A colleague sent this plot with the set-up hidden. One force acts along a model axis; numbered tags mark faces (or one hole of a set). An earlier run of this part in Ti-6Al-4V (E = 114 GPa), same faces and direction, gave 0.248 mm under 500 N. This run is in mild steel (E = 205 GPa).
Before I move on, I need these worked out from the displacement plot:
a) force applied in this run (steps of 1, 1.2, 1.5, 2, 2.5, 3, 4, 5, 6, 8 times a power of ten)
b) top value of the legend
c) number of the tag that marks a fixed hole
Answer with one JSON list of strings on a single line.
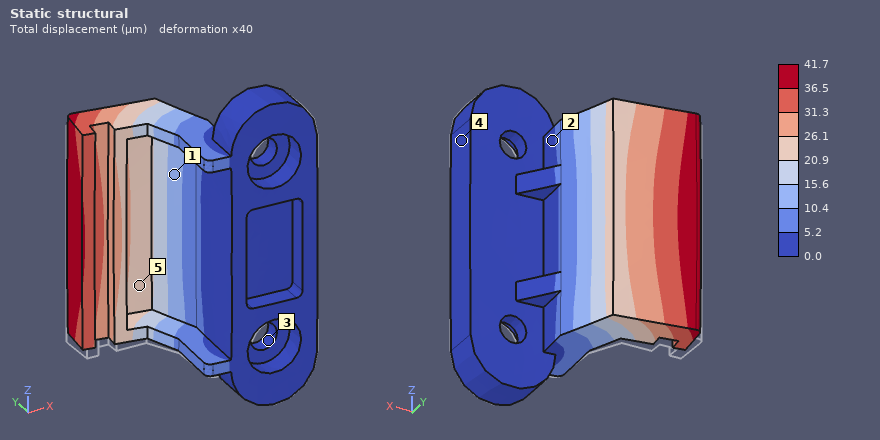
["150 N", "41.7 µm", "3"]
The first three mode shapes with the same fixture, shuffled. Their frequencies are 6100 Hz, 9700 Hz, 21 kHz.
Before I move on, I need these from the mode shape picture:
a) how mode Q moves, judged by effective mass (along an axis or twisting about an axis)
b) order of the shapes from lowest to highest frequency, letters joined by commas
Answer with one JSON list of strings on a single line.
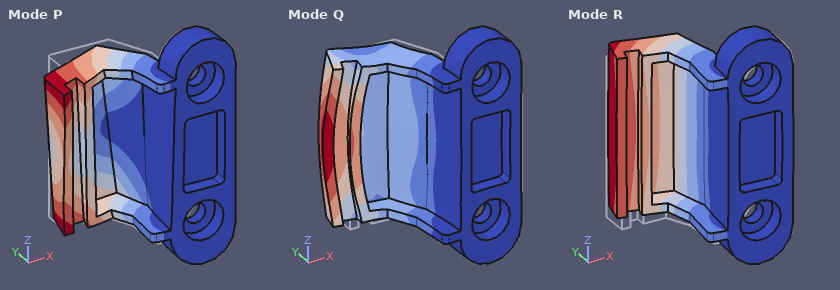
["along X", "R, P, Q"]
